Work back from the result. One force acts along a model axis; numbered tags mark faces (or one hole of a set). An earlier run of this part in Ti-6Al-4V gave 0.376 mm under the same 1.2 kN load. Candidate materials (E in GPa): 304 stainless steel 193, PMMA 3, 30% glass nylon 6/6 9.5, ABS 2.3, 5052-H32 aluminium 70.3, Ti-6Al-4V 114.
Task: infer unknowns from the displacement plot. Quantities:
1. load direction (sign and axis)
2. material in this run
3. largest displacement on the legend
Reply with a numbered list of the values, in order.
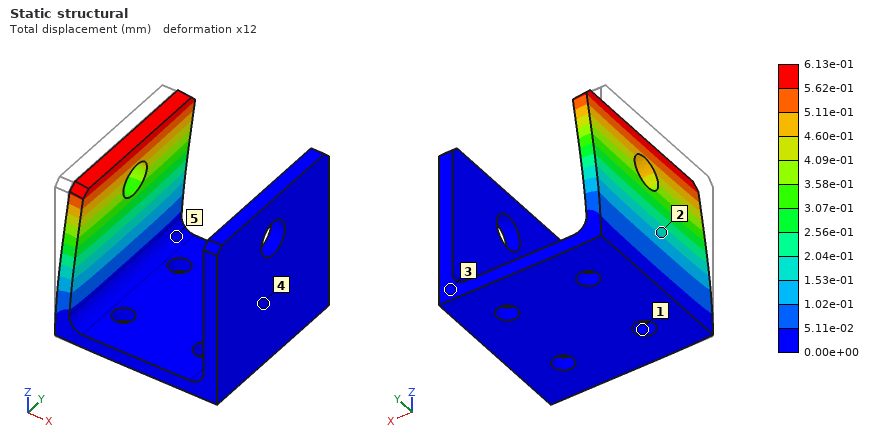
1. +X
2. 5052-H32 aluminium
3. 6.13e-01 mm
